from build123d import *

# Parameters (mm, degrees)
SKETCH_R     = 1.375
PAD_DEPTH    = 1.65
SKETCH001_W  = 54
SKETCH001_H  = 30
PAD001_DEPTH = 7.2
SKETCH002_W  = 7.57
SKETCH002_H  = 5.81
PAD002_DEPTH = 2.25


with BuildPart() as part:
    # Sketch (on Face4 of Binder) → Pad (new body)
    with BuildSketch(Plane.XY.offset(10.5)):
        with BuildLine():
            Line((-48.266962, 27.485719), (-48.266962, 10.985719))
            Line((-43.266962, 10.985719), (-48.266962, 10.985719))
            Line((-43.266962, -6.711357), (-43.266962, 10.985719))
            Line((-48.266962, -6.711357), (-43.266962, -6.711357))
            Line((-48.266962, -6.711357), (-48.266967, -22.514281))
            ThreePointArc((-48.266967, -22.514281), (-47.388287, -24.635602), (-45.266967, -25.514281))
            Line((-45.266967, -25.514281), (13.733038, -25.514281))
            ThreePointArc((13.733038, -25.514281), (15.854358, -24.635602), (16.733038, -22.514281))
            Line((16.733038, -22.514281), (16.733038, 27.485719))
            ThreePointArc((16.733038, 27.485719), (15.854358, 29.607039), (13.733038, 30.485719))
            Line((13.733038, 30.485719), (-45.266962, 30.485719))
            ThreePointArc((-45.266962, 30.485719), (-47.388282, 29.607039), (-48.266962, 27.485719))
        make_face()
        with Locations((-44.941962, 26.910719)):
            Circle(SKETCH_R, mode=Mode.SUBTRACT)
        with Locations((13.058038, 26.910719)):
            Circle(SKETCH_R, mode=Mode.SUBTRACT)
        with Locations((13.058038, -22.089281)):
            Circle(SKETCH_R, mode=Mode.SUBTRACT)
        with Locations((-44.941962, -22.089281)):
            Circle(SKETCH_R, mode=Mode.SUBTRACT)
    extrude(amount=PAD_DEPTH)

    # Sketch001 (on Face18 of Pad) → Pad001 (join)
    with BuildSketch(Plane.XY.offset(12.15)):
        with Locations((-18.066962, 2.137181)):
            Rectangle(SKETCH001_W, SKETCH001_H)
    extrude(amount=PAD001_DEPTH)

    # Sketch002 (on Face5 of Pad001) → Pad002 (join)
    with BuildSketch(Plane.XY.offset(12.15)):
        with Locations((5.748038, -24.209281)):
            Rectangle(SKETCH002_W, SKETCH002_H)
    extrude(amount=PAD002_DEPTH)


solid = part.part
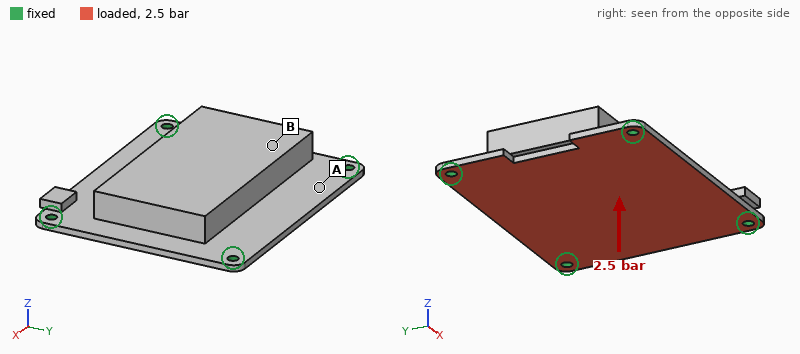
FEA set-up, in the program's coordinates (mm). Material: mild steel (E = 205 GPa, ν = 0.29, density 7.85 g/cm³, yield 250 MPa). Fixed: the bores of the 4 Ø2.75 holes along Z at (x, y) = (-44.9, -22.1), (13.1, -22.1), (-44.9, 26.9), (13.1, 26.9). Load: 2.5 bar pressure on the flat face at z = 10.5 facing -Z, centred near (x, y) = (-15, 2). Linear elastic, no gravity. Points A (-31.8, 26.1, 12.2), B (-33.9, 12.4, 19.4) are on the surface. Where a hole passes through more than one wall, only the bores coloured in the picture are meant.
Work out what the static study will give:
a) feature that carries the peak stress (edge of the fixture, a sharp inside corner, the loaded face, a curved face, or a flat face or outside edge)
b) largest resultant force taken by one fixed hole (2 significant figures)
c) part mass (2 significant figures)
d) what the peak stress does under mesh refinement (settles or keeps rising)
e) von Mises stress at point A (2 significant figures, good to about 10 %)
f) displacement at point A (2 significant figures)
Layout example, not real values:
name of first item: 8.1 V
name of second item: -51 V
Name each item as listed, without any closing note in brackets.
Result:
feature that carries the peak stress: edge of the fixture
largest resultant force taken by one fixed hole: 260 N
part mass: 140 g
what the peak stress does under mesh refinement: keeps rising
von Mises stress at point A: 34 MPa
displacement at point A: 21 µm
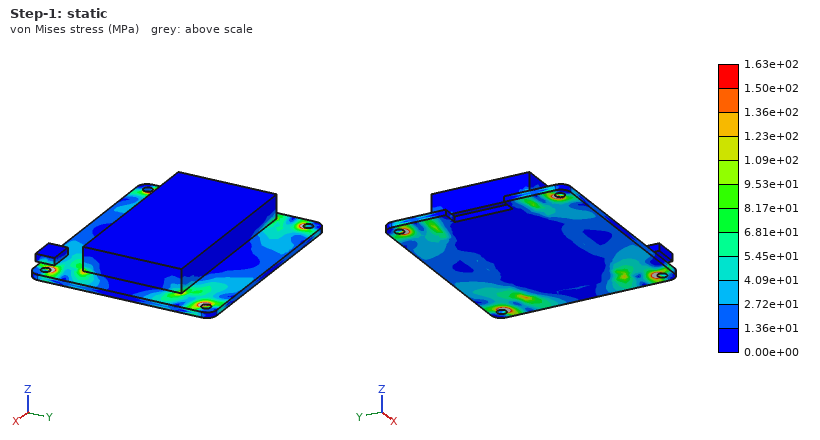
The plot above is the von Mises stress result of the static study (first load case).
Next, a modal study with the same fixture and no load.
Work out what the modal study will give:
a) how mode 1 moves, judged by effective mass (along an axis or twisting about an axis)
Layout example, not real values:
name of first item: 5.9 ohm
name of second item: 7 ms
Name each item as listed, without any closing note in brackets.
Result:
how mode 1 moves, judged by effective mass: along Z
